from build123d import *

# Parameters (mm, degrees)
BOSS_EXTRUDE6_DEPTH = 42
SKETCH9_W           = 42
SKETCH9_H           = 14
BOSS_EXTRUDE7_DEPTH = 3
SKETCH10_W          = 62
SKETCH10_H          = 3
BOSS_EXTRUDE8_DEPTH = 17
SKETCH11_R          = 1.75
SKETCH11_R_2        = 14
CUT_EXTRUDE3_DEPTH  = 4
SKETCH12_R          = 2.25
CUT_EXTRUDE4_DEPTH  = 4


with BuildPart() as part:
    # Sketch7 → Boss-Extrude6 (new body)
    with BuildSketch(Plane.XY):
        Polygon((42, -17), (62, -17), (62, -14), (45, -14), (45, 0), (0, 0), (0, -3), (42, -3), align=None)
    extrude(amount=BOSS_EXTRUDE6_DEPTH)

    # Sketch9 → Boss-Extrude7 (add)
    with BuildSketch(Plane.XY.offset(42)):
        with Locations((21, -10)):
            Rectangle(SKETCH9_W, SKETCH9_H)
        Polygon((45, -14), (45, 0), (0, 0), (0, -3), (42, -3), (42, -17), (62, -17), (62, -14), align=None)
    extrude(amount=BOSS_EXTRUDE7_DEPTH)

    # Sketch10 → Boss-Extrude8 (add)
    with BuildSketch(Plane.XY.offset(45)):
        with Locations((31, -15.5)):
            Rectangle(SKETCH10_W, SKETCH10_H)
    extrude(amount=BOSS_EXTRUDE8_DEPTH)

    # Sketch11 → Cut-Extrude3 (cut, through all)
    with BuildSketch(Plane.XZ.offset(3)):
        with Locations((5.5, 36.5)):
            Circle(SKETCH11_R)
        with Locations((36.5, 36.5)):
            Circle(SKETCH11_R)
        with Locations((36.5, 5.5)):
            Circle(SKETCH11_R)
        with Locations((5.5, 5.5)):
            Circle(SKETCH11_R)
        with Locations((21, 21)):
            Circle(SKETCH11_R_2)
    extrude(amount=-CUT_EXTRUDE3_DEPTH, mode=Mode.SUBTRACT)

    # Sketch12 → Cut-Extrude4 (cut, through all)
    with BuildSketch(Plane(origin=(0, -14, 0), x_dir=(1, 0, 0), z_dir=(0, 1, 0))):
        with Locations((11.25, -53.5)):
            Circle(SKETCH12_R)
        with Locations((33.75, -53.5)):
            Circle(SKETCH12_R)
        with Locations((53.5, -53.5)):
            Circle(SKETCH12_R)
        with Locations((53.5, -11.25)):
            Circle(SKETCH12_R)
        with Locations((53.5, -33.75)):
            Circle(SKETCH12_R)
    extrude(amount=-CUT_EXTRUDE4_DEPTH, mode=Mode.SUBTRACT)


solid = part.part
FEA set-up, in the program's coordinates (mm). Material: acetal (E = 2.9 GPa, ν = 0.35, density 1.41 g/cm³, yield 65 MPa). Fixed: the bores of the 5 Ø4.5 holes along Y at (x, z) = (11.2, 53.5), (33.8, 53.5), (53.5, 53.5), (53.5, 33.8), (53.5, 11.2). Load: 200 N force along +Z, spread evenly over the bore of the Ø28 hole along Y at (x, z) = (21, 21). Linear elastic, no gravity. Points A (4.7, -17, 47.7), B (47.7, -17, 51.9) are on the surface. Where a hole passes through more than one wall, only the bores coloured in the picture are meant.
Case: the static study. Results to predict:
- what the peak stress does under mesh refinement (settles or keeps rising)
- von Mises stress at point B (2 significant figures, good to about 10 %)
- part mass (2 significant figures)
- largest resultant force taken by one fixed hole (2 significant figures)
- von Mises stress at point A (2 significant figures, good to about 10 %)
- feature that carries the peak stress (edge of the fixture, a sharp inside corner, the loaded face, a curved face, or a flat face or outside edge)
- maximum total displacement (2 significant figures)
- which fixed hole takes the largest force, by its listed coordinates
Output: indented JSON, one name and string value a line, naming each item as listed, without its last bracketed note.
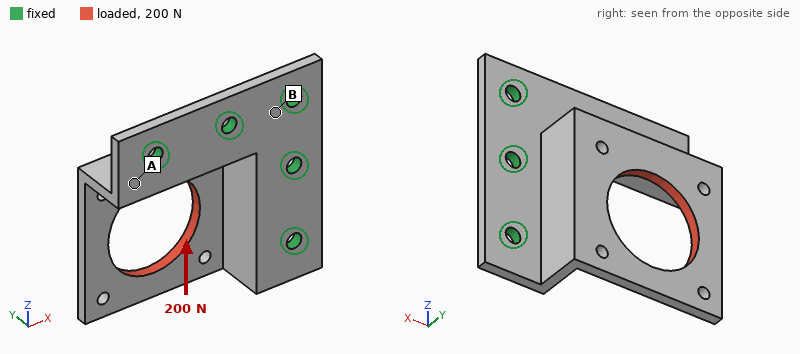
{
  "what the peak stress does under mesh refinement": "keeps rising",
  "von Mises stress at point B": "2.8 MPa",
  "part mass": "18 g",
  "largest resultant force taken by one fixed hole": "120 N",
  "von Mises stress at point A": "11 MPa",
  "feature that carries the peak stress": "edge of the fixture",
  "maximum total displacement": "0.83 mm",
  "which fixed hole takes the largest force, by its listed coordinates": "(53.5, 11.2)"
}
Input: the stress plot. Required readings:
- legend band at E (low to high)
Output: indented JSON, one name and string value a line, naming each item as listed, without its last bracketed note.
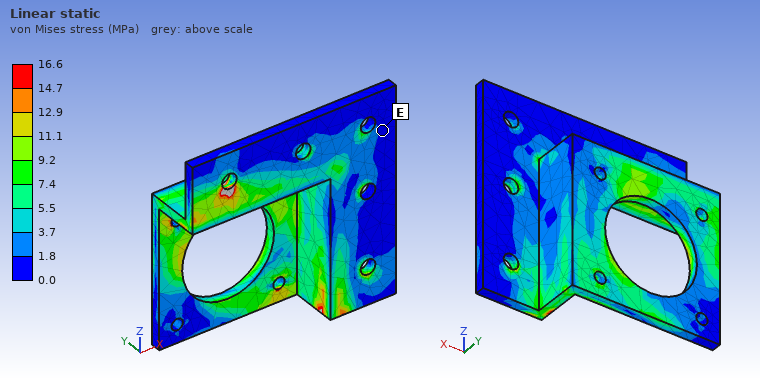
{
  "legend band at E": "0.0 to 1.8 MPa"
}
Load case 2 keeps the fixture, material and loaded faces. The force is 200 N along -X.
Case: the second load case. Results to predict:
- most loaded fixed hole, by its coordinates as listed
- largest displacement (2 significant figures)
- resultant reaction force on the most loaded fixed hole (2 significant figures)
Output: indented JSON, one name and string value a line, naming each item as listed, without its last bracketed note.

{
  "most loaded fixed hole, by its coordinates as listed": "(11.2, 53.5)",
  "largest displacement": "0.83 mm",
  "resultant reaction force on the most loaded fixed hole": "120 N"
}
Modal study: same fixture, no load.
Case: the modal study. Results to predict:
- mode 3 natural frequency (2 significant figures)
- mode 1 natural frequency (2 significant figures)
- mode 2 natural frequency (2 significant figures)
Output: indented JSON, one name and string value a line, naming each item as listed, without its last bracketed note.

{
  "mode 3 natural frequency": "1700 Hz",
  "mode 1 natural frequency": "560 Hz",
  "mode 2 natural frequency": "990 Hz"
}
